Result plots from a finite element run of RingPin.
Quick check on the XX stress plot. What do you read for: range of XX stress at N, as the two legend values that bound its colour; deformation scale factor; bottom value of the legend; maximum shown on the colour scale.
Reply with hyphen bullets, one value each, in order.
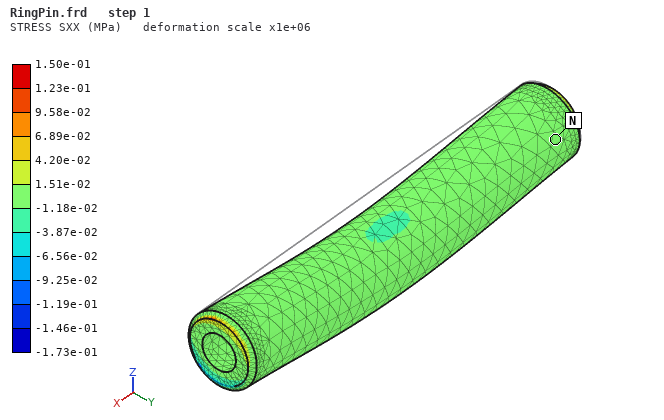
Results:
- -1.18e-02 to 1.51e-02 MPa
- 1e+06
- -1.73e-01 MPa
- 1.50e-01 MPa
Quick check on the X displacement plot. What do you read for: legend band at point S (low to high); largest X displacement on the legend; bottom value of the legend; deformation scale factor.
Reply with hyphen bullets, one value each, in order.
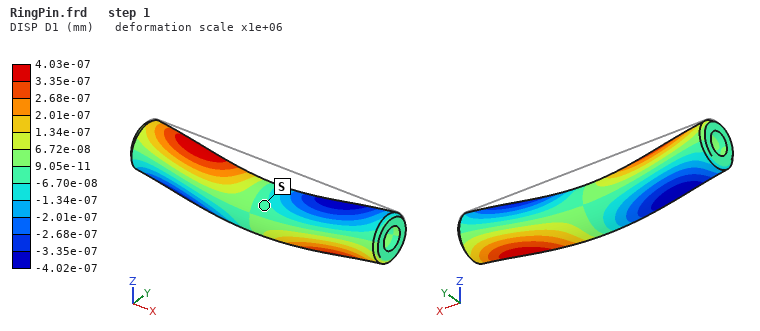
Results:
- -6.70e-08 to 9.05e-11 mm
- 4.03e-07 mm
- -4.02e-07 mm
- 1e+06
